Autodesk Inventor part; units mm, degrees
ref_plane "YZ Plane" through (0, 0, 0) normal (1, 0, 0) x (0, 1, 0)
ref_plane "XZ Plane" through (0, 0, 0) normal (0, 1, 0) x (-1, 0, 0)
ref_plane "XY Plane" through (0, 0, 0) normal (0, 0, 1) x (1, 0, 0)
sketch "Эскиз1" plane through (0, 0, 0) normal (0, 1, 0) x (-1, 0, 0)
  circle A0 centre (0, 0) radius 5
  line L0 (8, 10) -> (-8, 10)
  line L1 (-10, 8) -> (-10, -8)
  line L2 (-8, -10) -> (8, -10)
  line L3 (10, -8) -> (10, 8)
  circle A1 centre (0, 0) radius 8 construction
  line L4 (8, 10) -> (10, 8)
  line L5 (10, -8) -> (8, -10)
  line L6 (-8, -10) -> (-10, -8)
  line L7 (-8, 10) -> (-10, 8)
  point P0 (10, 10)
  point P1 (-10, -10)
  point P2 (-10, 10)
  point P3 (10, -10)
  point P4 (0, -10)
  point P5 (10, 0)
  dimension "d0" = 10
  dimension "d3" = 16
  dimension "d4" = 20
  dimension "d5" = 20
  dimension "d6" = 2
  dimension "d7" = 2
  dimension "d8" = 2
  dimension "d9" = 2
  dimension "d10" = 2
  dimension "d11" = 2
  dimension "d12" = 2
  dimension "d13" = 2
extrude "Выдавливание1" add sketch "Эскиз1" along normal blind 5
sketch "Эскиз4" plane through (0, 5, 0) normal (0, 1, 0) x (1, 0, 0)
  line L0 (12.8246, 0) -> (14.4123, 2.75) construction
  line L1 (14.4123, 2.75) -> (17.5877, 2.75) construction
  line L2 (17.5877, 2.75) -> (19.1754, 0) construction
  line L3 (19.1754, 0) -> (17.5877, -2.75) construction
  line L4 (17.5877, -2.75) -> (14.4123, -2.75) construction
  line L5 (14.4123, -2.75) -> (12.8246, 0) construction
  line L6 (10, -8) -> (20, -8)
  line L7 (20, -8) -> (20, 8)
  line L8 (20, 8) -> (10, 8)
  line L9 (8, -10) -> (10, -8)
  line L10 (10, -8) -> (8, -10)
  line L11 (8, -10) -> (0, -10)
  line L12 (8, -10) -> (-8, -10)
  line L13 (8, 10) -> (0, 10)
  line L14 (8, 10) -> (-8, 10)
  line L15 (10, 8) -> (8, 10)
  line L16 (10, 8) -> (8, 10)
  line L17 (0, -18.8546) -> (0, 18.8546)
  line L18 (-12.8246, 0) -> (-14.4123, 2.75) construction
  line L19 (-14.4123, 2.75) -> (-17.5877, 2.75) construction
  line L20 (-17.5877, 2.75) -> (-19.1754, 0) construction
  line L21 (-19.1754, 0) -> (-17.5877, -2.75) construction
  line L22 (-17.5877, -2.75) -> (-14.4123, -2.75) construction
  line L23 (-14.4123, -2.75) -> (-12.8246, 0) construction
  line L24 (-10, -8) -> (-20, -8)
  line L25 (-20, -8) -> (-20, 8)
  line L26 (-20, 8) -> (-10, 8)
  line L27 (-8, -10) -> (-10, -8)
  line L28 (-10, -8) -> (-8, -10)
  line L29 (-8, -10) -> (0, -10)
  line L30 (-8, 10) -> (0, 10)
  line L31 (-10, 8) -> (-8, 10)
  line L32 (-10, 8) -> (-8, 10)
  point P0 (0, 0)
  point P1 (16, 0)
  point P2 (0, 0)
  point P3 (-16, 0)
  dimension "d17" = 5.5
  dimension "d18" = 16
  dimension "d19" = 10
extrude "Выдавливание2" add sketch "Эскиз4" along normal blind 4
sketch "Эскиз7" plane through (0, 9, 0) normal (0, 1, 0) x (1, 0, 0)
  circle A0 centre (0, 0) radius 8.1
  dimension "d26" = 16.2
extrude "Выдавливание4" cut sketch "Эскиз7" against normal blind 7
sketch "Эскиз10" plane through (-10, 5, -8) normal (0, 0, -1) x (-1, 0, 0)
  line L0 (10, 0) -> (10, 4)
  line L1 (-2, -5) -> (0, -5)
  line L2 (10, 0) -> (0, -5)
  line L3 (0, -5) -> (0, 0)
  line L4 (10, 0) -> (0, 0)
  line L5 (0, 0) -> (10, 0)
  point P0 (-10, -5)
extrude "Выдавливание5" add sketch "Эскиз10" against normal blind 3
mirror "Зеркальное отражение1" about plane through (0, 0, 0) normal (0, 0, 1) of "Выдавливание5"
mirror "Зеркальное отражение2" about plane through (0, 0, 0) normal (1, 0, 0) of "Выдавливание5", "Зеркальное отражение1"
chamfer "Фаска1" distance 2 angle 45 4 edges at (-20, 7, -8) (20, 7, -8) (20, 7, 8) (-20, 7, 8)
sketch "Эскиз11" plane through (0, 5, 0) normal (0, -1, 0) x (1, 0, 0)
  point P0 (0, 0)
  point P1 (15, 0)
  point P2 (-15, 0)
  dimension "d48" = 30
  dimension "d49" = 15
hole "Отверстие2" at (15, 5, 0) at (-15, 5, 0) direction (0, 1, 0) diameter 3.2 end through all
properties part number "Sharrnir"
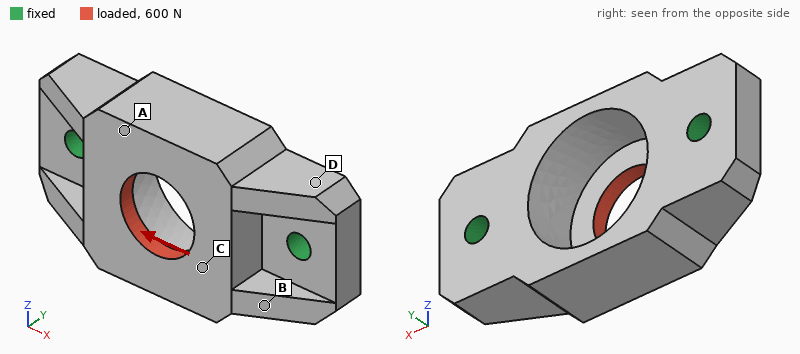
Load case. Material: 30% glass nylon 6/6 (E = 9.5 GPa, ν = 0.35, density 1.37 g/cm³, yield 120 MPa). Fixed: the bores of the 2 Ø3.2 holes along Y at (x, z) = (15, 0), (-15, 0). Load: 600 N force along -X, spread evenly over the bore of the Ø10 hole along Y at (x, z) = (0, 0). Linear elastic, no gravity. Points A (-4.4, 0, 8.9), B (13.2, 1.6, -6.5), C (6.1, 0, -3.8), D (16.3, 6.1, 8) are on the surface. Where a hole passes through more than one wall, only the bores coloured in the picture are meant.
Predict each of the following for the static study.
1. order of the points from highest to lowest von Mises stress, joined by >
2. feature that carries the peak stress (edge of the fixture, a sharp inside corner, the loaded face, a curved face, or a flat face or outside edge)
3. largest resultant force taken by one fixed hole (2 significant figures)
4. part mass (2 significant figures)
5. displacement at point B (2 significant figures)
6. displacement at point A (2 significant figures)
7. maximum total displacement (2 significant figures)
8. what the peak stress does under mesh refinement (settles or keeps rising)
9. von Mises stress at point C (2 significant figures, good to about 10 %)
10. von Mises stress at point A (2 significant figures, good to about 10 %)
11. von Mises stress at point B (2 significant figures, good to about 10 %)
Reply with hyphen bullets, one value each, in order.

- C > B > A > D
- edge of the fixture
- 320 N
- 4.7 g
- 14 µm
- 14 µm
- 30 µm
- keeps rising
- 13 MPa
- 2.8 MPa
- 5.5 MPa
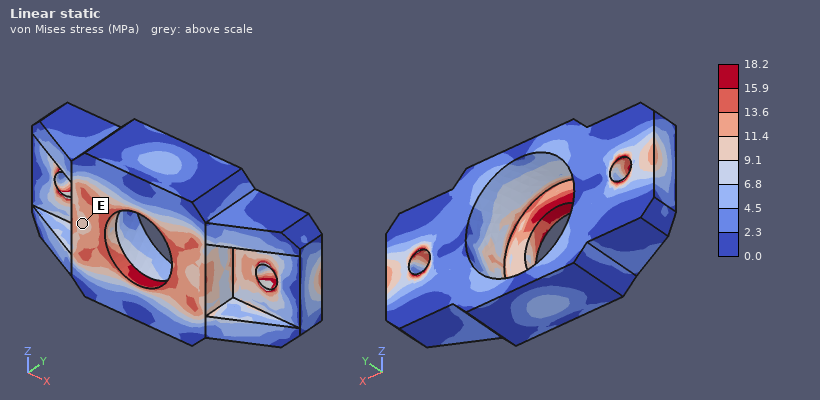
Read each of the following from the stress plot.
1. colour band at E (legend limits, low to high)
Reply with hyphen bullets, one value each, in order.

- 9.1 to 11.4 MPa
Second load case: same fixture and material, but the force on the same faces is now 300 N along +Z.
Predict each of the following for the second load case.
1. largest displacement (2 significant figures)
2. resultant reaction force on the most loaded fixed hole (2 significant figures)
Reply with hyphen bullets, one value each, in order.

- 63 µm
- 150 N
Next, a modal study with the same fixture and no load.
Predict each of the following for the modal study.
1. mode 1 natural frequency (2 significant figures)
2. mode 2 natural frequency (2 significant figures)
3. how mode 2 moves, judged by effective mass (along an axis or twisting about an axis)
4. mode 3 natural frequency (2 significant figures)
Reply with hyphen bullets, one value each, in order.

- 7500 Hz
- 12 kHz
- along Y
- 16 kHz
